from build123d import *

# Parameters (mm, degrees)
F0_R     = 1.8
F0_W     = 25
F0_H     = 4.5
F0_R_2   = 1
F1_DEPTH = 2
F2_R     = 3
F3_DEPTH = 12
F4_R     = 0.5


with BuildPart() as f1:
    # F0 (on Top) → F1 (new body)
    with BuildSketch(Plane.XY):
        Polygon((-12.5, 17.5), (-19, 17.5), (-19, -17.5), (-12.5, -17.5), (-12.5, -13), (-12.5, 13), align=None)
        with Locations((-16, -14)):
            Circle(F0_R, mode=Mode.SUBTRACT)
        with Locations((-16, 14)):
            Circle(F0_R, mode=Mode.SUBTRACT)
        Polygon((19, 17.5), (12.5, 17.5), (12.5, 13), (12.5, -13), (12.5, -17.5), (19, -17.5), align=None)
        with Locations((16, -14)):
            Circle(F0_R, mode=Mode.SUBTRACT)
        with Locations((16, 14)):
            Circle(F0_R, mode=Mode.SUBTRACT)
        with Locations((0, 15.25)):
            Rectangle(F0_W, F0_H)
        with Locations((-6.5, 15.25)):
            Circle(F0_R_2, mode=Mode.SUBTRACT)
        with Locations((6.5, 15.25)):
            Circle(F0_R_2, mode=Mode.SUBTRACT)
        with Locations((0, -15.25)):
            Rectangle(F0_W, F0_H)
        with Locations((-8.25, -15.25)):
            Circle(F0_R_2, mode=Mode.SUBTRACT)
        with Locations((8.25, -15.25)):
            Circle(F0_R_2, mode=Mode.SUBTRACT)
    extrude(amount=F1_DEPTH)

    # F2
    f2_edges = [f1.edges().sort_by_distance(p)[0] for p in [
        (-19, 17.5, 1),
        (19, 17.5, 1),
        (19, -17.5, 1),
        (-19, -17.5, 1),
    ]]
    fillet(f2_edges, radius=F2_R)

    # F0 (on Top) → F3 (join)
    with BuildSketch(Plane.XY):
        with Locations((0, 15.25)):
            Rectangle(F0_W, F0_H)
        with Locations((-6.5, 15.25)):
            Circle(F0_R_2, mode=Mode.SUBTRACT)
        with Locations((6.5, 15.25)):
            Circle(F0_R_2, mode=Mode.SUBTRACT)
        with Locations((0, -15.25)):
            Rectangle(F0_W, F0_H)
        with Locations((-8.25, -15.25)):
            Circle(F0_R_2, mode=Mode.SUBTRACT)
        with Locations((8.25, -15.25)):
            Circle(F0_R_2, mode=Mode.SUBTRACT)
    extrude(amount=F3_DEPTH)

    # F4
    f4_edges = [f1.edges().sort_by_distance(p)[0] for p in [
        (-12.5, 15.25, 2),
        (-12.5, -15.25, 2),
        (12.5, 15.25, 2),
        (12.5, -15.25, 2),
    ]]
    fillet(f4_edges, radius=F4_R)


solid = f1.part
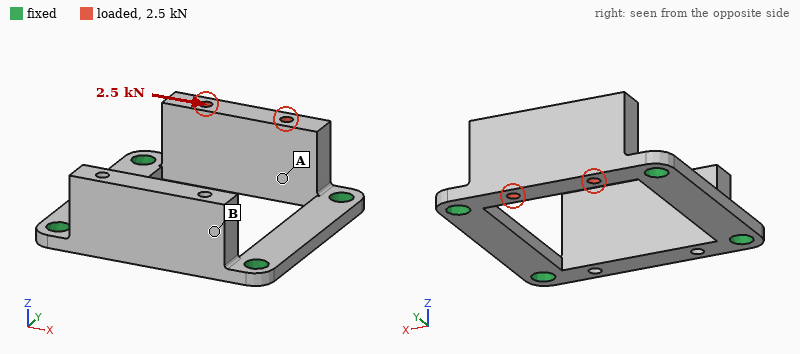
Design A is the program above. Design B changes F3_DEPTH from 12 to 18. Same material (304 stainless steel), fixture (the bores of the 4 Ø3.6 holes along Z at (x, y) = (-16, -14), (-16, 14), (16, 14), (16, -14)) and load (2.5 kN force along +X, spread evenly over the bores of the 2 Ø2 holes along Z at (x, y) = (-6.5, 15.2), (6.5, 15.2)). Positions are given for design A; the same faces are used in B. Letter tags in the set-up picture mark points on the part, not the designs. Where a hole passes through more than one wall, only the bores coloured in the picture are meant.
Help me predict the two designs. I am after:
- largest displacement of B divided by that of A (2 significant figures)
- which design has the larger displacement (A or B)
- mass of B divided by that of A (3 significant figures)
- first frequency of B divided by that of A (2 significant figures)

1.7
B
1.38
0.53
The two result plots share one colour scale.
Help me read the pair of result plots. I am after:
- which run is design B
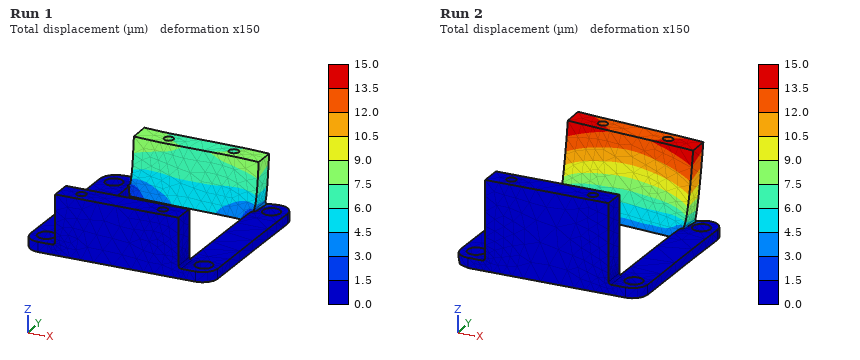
Run 2
